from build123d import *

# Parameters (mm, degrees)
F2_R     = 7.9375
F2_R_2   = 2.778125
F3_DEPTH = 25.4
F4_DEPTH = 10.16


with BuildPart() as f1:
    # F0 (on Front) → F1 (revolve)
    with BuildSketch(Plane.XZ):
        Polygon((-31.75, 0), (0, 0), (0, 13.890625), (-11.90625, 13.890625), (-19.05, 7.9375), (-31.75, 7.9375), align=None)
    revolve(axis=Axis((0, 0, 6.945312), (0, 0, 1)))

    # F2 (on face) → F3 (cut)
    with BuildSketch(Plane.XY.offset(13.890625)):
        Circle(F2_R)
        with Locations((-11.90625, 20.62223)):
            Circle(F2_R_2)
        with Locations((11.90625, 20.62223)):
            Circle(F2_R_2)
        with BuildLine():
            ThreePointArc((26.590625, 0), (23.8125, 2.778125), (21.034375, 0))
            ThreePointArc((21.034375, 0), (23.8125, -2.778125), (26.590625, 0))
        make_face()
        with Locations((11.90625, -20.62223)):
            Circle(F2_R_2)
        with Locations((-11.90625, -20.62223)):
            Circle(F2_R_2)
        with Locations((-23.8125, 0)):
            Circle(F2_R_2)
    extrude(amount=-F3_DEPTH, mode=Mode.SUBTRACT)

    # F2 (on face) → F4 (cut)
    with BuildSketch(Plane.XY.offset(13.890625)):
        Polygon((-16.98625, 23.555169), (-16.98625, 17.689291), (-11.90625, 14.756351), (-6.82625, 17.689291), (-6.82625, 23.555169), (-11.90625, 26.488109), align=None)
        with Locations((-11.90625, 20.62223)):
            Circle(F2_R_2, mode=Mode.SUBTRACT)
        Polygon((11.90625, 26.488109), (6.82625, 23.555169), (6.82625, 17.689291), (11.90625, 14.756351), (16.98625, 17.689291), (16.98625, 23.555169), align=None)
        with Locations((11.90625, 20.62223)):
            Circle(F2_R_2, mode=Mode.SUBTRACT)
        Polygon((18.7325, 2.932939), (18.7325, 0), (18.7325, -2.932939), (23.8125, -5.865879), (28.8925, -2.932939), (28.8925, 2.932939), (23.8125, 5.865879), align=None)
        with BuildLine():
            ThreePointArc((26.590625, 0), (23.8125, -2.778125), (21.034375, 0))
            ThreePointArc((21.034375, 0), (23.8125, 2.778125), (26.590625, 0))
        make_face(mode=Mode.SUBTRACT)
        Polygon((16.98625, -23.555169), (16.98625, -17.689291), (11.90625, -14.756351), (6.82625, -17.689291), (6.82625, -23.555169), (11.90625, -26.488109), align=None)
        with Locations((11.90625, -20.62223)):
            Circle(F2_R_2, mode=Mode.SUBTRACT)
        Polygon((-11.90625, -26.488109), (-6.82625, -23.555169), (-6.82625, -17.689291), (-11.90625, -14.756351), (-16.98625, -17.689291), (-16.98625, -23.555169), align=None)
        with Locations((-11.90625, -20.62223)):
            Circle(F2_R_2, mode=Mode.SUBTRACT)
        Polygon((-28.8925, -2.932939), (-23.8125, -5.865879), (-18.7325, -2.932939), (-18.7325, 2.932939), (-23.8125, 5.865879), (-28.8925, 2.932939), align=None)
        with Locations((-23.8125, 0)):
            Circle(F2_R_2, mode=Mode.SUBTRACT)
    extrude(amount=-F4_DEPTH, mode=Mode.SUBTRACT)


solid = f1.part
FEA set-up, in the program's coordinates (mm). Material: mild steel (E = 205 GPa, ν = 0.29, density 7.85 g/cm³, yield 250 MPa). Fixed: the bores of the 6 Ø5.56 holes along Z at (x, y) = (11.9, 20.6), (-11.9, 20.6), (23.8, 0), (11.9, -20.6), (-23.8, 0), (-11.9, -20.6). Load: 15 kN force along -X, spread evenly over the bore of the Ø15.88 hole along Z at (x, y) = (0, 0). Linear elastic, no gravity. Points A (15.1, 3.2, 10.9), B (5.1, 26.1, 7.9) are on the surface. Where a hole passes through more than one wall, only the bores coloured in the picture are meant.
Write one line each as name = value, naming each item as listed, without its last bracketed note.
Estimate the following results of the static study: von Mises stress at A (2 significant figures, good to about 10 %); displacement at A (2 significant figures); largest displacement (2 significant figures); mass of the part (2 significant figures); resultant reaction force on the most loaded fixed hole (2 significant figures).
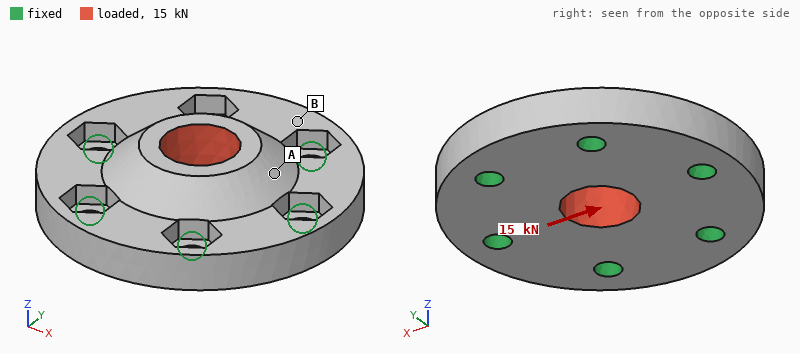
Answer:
von Mises stress at A = 25 MPa
displacement at A = 3.8 µm
largest displacement = 5.2 µm
mass of the part = 190 g
resultant reaction force on the most loaded fixed hole = 3.6 kN
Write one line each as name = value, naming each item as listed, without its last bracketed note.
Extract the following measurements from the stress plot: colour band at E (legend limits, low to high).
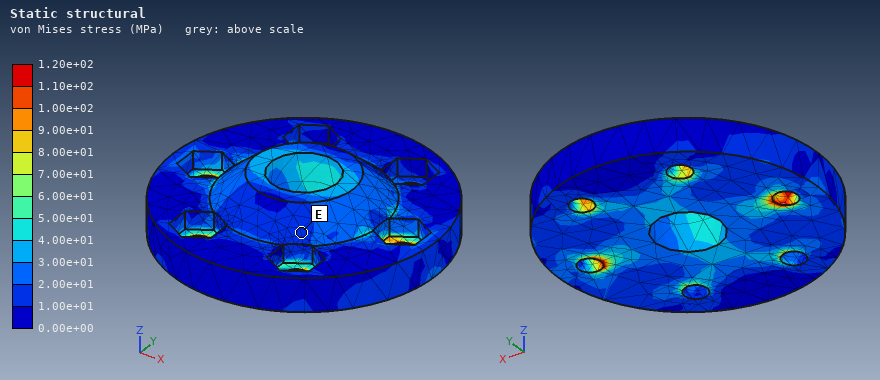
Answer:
colour band at E = 1.00e+01 to 2.00e+01 MPa
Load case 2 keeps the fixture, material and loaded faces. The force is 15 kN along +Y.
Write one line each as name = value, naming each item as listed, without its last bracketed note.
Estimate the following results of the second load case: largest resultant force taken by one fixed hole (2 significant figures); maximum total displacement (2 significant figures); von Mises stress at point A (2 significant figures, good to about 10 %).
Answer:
largest resultant force taken by one fixed hole = 3.2 kN
maximum total displacement = 5.2 µm
von Mises stress at point A = 13 MPa
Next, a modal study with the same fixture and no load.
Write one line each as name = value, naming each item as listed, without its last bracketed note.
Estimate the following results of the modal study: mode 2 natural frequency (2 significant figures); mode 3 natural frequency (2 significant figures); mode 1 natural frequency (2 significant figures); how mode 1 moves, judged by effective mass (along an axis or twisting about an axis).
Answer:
mode 2 natural frequency = 29 kHz
mode 3 natural frequency = 29 kHz
mode 1 natural frequency = 25 kHz
how mode 1 moves, judged by effective mass = along Z
